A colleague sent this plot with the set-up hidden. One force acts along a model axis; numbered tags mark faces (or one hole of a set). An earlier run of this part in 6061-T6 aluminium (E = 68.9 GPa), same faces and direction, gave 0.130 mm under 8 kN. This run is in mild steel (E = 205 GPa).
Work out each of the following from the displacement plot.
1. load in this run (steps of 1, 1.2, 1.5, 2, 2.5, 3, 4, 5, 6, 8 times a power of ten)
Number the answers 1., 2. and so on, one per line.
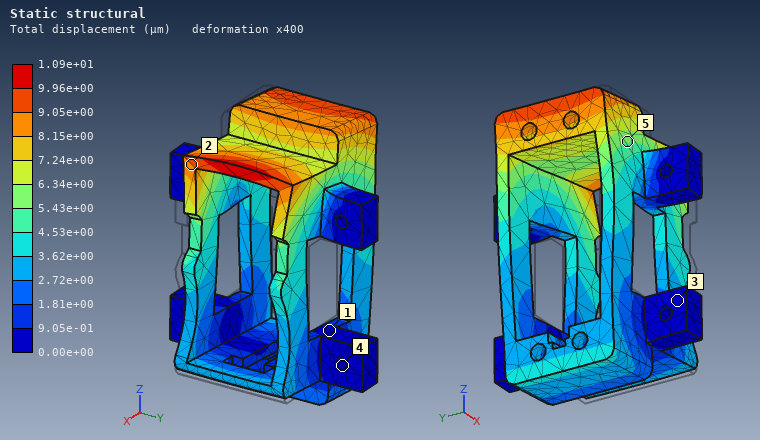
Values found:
1. 2 kN
